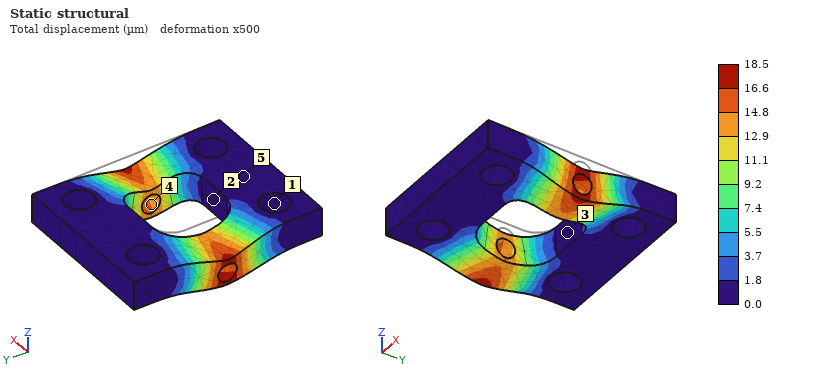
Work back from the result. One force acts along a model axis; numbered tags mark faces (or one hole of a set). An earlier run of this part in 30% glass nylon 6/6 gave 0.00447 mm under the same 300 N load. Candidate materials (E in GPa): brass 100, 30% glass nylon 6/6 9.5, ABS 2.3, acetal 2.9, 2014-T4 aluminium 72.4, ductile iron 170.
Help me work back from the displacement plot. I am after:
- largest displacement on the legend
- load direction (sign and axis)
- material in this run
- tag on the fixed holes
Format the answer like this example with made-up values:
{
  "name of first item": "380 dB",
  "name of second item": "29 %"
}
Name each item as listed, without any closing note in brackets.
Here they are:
{
  "largest displacement on the legend": "18.5 µm",
  "load direction": "-Z",
  "material in this run": "ABS",
  "tag on the fixed holes": "1"
}
